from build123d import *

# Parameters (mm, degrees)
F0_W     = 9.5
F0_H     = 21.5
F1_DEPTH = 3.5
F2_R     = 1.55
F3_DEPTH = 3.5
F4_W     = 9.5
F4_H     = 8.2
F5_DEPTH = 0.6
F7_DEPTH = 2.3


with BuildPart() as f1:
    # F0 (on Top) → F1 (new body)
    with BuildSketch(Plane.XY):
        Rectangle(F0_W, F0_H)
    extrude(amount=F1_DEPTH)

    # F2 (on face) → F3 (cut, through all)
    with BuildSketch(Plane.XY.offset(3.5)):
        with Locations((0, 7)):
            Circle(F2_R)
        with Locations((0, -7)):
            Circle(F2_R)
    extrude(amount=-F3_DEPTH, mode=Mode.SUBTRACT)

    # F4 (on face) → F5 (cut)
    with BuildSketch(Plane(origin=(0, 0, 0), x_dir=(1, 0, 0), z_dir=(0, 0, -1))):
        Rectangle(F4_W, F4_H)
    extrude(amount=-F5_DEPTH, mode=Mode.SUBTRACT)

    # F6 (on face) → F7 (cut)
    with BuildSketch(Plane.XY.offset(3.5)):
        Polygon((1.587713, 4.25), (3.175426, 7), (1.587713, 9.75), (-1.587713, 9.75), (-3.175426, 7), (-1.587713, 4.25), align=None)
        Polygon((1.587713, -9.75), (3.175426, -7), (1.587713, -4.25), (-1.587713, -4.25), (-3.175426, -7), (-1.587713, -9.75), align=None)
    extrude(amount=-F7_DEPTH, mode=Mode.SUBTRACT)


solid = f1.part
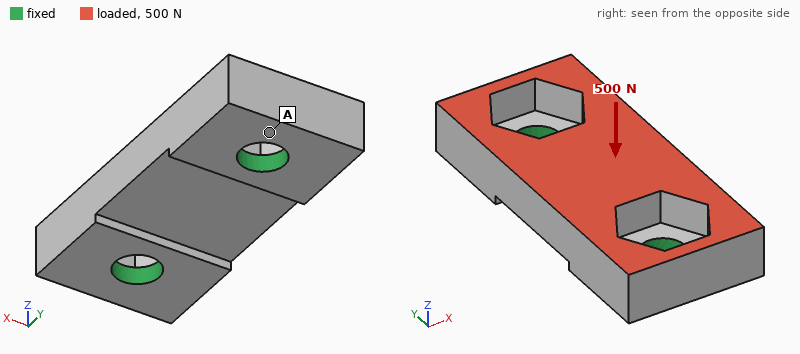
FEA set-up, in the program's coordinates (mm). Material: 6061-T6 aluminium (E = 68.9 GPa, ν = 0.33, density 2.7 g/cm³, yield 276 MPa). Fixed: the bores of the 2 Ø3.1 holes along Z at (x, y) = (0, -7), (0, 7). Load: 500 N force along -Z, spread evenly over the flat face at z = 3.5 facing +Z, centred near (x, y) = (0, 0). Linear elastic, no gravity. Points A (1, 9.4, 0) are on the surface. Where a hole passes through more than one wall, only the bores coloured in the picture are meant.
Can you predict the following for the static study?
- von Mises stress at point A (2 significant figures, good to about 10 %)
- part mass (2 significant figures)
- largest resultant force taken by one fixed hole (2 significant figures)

16 MPa
1.4 g
280 N
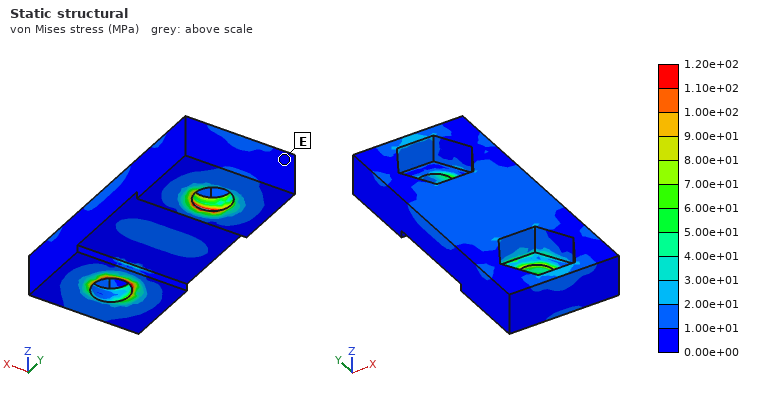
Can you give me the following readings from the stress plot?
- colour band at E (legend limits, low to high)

0.00e+00 to 1.00e+01 MPa
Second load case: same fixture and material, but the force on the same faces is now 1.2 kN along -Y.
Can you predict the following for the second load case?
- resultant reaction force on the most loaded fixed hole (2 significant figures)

640 N
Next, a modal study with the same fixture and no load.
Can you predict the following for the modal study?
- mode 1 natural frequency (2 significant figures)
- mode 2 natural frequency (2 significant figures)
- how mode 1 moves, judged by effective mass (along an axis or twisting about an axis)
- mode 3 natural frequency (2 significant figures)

31 kHz
49 kHz
along X
50 kHz
